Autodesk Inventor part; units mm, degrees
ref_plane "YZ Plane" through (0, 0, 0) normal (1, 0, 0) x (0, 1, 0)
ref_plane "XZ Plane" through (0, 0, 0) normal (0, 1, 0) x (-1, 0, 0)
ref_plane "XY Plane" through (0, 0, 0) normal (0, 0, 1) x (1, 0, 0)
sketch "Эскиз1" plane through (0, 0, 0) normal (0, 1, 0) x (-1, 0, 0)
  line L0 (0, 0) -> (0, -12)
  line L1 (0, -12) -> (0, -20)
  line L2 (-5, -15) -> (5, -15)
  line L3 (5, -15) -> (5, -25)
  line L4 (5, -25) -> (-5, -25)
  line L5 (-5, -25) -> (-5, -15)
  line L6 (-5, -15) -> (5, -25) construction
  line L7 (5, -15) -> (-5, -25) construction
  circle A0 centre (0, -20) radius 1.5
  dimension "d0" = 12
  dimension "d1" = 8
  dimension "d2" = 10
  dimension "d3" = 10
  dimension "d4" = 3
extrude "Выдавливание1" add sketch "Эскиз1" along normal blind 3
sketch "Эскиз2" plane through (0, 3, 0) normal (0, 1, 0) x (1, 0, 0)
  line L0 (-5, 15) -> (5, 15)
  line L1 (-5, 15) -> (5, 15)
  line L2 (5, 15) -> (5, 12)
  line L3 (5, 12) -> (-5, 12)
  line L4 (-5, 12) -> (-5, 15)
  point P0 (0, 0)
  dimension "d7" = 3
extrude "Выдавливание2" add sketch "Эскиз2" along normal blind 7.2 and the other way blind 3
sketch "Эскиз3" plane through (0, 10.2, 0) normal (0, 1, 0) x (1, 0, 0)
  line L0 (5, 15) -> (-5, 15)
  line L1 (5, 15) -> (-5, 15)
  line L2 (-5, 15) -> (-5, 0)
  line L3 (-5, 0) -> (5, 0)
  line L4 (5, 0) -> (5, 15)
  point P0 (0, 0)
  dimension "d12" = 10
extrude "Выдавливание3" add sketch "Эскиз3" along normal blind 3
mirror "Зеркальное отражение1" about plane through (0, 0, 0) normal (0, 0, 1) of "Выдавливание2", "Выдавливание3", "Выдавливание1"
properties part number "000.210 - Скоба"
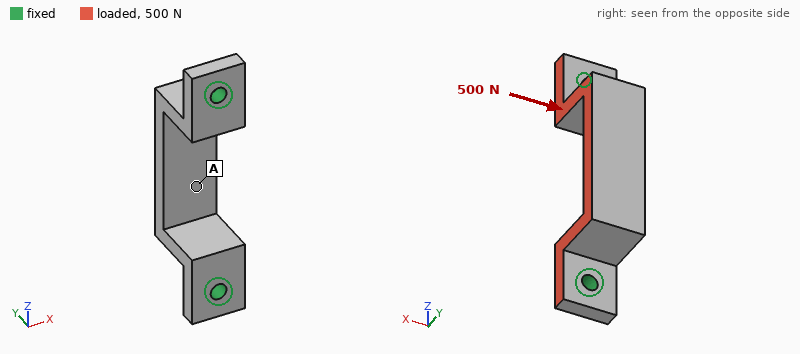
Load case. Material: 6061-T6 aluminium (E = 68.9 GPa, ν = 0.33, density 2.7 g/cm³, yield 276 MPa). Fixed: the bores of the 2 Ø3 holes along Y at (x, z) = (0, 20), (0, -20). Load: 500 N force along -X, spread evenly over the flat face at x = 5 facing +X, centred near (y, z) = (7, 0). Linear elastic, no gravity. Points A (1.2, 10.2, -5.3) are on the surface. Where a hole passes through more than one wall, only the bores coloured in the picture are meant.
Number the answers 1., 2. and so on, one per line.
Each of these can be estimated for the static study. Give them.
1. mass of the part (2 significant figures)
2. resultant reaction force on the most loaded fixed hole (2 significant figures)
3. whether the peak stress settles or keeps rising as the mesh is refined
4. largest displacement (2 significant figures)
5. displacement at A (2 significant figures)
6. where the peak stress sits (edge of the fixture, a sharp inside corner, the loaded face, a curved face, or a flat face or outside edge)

1. 5.6 g
2. 250 N
3. keeps rising
4. 48 µm
5. 36 µm
6. edge of the fixture
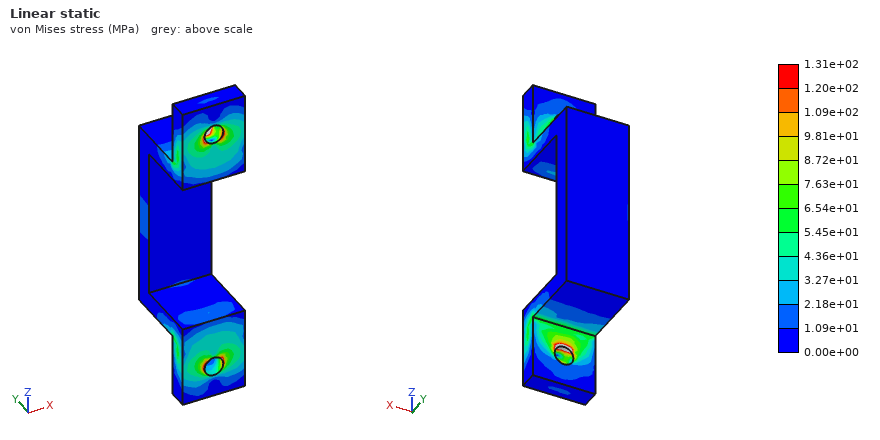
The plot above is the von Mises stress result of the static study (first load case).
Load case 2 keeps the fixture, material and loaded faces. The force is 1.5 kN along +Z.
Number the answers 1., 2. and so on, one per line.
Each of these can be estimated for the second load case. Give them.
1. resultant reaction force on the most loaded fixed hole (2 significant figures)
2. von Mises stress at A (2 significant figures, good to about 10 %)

1. 780 N
2. 68 MPa
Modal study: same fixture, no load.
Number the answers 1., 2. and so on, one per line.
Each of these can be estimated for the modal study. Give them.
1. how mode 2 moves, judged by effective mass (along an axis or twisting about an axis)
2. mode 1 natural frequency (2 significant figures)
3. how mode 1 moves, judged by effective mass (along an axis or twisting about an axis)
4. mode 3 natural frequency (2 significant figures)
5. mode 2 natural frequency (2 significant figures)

1. along Z
2. 7600 Hz
3. along X
4. 14 kHz
5. 10000 Hz
